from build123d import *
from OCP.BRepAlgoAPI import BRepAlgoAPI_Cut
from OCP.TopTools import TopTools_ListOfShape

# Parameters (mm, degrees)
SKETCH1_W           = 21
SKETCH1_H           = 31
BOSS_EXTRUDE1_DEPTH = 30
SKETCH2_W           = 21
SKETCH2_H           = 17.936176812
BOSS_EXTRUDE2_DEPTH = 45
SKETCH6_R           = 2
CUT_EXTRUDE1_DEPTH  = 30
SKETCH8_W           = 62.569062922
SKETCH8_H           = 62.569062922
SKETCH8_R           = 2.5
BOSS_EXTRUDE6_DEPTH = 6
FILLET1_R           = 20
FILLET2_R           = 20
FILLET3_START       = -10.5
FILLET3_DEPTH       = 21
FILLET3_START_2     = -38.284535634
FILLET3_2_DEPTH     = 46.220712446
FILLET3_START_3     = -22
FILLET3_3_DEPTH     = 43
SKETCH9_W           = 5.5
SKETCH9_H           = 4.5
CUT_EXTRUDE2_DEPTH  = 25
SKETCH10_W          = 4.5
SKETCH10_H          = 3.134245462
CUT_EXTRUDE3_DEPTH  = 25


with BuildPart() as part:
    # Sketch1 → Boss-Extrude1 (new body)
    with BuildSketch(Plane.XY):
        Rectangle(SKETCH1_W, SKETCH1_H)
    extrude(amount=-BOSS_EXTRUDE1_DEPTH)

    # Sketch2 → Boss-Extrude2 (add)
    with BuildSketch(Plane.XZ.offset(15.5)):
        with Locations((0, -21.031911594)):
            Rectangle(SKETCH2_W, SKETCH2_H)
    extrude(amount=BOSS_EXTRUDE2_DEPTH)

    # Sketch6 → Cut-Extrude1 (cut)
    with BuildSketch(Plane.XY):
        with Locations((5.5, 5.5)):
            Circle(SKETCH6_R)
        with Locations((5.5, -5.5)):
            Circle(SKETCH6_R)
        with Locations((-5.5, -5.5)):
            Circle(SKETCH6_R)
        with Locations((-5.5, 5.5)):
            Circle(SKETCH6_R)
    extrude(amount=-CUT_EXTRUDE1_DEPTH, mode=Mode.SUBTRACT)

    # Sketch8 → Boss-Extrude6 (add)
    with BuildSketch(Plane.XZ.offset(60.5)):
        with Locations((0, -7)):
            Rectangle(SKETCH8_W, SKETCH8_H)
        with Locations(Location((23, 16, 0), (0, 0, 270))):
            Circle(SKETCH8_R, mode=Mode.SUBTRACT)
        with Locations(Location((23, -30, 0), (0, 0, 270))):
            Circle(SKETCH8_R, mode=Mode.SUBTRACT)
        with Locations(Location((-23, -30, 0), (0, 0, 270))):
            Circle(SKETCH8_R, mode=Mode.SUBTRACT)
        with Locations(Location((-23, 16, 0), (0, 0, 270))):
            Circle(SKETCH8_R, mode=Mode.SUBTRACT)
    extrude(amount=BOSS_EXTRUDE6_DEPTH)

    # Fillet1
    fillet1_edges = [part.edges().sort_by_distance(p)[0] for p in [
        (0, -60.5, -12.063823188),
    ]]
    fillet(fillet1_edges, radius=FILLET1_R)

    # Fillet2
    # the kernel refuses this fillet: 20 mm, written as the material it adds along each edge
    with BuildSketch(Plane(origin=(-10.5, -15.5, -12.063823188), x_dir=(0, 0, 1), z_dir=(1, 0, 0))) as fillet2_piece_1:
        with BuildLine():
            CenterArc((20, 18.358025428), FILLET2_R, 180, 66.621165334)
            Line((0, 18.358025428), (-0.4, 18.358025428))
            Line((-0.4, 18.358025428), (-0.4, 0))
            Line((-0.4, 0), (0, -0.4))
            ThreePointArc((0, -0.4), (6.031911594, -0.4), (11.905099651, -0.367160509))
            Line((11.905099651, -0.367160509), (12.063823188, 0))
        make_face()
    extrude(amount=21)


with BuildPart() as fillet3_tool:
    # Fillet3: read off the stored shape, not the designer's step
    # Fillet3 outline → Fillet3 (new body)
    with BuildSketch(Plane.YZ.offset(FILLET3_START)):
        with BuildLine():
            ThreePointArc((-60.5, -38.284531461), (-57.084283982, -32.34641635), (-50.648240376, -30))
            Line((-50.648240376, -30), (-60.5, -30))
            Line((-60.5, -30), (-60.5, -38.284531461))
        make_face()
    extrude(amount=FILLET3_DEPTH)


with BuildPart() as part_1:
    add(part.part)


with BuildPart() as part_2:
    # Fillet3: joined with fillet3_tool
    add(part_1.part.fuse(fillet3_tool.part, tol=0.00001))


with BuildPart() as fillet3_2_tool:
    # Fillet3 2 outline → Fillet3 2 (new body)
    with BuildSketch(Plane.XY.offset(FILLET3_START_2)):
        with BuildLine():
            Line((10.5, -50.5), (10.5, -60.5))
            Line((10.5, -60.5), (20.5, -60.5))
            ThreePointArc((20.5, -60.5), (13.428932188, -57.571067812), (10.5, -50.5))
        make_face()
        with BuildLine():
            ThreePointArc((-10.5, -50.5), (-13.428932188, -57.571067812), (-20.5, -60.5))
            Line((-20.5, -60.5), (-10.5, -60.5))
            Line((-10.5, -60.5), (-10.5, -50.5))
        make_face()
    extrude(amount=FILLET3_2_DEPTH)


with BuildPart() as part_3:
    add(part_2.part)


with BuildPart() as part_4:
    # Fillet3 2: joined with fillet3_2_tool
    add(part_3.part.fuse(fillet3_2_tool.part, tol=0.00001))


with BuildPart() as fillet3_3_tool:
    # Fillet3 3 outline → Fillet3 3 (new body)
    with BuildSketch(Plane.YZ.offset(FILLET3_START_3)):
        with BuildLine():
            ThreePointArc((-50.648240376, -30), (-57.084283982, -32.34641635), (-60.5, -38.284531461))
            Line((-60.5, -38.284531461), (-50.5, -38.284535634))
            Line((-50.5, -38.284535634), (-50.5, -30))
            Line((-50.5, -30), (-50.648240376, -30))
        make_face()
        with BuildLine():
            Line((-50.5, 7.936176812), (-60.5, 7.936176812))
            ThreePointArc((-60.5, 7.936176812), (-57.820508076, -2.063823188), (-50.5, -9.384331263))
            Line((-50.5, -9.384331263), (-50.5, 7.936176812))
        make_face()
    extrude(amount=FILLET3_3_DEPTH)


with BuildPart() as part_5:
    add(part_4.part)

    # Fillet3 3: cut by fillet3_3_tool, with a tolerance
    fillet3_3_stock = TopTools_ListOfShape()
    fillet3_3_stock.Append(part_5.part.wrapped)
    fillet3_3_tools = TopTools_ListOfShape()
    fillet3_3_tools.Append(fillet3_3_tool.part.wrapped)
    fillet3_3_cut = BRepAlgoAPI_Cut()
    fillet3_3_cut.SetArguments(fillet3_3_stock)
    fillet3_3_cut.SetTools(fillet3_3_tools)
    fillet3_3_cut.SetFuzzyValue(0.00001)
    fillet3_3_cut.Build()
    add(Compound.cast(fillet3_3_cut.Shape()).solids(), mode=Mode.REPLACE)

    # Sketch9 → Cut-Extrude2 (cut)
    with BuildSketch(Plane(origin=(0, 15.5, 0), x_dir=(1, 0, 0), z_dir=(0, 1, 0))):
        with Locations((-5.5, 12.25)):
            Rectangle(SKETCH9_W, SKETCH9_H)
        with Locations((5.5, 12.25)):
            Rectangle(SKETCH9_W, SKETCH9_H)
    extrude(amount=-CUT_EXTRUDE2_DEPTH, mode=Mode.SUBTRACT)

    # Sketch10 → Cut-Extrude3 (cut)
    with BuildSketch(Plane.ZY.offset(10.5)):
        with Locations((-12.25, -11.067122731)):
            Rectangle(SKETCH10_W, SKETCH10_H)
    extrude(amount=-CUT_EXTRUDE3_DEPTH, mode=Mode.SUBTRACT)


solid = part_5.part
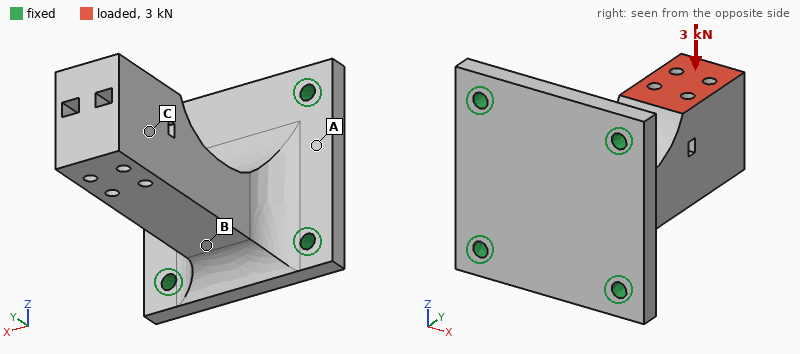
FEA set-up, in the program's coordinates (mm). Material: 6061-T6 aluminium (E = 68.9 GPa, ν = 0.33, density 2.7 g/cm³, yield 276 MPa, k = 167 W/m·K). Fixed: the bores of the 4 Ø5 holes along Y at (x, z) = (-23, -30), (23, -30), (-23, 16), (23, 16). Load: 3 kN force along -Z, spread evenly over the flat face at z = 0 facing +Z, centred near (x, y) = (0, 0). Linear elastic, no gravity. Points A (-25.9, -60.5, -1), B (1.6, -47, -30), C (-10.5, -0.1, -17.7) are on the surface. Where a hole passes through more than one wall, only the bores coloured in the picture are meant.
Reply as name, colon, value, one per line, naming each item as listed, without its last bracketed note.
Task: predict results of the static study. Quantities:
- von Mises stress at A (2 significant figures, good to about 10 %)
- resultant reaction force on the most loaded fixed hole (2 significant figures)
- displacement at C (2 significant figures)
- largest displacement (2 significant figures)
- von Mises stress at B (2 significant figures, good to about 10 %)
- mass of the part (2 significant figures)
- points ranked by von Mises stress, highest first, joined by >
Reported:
von Mises stress at A: 41 MPa
resultant reaction force on the most loaded fixed hole: 2.5 kN
displacement at C: 0.44 mm
largest displacement: 0.61 mm
von Mises stress at B: 100 MPa
mass of the part: 170 g
points ranked by von Mises stress, highest first, joined by >: B > A > C
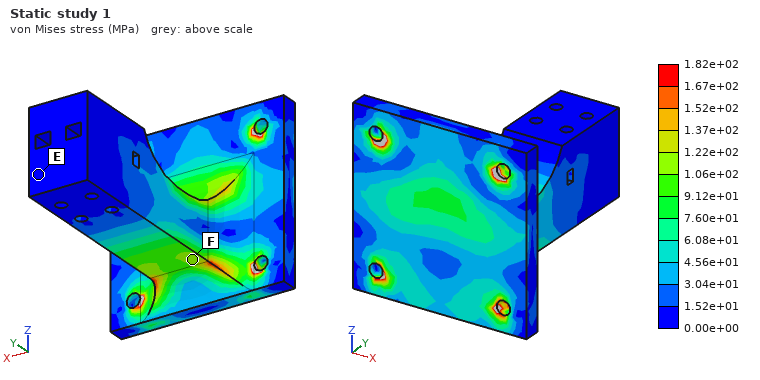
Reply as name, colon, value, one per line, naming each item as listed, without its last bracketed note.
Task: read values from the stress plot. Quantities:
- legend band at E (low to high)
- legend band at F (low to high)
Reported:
legend band at E: 0.00e+00 to 1.52e+01 MPa
legend band at F: 1.06e+02 to 1.22e+02 MPa
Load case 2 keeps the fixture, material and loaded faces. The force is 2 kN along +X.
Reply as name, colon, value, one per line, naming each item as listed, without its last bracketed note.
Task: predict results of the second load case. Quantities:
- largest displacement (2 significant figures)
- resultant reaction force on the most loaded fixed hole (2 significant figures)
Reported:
largest displacement: 0.36 mm
resultant reaction force on the most loaded fixed hole: 2.9 kN
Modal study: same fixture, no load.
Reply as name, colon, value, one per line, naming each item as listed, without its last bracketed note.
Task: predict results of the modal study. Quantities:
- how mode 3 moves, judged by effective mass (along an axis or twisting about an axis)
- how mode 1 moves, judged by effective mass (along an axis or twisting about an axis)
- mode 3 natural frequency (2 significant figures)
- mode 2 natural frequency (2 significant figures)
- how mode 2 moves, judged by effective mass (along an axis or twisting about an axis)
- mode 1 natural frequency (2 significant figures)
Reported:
how mode 3 moves, judged by effective mass: along Y
how mode 1 moves, judged by effective mass: along Z
mode 3 natural frequency: 6600 Hz
mode 2 natural frequency: 2100 Hz
how mode 2 moves, judged by effective mass: along X
mode 1 natural frequency: 1700 Hz
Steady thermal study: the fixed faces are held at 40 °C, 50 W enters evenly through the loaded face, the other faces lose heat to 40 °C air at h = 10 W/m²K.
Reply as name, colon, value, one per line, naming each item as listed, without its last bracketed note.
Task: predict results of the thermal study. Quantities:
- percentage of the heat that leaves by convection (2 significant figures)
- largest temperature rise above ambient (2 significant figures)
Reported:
percentage of the heat that leaves by convection: 7.6 %
largest temperature rise above ambient: 55 K
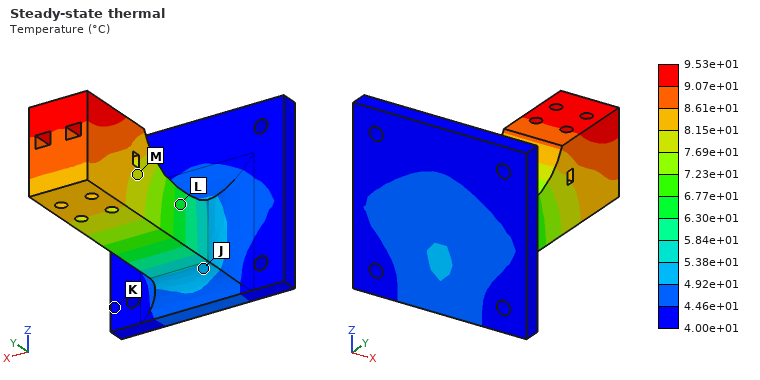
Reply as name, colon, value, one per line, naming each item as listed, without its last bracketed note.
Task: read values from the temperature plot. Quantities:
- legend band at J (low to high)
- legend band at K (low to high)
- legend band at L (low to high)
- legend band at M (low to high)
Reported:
legend band at J: 4.92e+01 to 5.38e+01 °C
legend band at K: 4.00e+01 to 4.46e+01 °C
legend band at L: 6.30e+01 to 6.77e+01 °C
legend band at M: 7.69e+01 to 8.15e+01 °C
